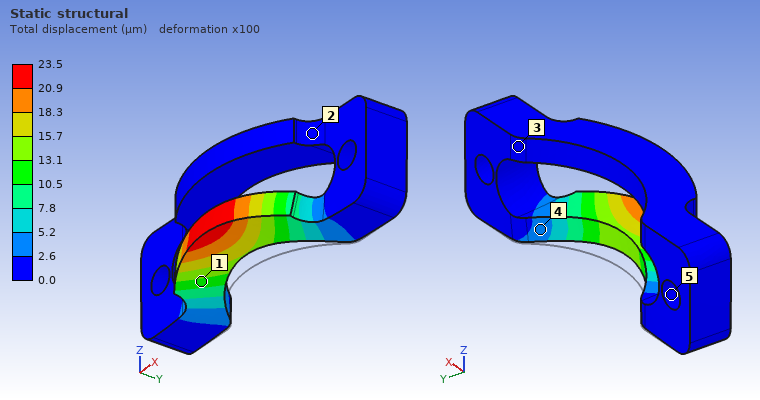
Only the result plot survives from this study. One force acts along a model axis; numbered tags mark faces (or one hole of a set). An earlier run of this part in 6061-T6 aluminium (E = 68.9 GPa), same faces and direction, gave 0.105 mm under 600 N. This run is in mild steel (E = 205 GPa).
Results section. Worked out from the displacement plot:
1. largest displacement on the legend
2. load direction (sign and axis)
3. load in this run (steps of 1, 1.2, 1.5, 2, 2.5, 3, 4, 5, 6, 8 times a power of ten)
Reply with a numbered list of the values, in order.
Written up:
1. 23.5 µm
2. +Z
3. 400 N
